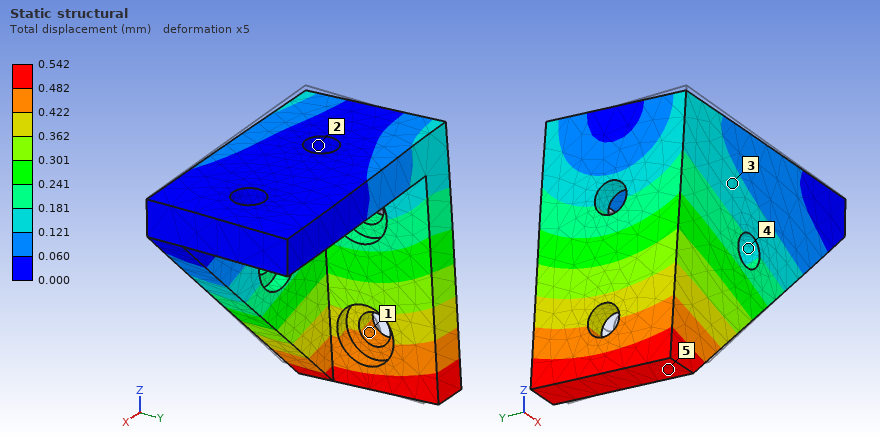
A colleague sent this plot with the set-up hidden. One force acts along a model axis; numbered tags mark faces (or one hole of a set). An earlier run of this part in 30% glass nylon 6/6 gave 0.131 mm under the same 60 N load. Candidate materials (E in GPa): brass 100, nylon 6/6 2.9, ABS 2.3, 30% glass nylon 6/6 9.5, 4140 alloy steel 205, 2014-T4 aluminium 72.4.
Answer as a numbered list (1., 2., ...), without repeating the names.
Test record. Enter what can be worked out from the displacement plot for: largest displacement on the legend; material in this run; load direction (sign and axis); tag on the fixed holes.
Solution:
1. 0.542 mm
2. ABS
3. +Y
4. 2
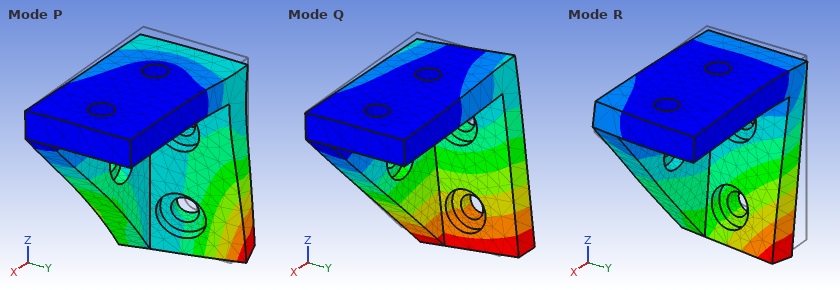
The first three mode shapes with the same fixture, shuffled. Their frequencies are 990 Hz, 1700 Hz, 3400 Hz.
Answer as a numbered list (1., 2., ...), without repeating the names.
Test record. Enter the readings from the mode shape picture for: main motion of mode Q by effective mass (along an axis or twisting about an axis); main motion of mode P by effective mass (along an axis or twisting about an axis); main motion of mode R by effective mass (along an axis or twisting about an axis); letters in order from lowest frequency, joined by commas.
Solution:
1. along Y
2. along Z
3. along X
4. Q, R, P
